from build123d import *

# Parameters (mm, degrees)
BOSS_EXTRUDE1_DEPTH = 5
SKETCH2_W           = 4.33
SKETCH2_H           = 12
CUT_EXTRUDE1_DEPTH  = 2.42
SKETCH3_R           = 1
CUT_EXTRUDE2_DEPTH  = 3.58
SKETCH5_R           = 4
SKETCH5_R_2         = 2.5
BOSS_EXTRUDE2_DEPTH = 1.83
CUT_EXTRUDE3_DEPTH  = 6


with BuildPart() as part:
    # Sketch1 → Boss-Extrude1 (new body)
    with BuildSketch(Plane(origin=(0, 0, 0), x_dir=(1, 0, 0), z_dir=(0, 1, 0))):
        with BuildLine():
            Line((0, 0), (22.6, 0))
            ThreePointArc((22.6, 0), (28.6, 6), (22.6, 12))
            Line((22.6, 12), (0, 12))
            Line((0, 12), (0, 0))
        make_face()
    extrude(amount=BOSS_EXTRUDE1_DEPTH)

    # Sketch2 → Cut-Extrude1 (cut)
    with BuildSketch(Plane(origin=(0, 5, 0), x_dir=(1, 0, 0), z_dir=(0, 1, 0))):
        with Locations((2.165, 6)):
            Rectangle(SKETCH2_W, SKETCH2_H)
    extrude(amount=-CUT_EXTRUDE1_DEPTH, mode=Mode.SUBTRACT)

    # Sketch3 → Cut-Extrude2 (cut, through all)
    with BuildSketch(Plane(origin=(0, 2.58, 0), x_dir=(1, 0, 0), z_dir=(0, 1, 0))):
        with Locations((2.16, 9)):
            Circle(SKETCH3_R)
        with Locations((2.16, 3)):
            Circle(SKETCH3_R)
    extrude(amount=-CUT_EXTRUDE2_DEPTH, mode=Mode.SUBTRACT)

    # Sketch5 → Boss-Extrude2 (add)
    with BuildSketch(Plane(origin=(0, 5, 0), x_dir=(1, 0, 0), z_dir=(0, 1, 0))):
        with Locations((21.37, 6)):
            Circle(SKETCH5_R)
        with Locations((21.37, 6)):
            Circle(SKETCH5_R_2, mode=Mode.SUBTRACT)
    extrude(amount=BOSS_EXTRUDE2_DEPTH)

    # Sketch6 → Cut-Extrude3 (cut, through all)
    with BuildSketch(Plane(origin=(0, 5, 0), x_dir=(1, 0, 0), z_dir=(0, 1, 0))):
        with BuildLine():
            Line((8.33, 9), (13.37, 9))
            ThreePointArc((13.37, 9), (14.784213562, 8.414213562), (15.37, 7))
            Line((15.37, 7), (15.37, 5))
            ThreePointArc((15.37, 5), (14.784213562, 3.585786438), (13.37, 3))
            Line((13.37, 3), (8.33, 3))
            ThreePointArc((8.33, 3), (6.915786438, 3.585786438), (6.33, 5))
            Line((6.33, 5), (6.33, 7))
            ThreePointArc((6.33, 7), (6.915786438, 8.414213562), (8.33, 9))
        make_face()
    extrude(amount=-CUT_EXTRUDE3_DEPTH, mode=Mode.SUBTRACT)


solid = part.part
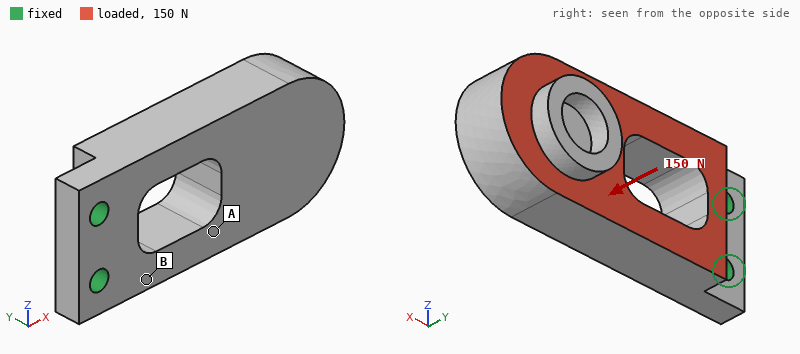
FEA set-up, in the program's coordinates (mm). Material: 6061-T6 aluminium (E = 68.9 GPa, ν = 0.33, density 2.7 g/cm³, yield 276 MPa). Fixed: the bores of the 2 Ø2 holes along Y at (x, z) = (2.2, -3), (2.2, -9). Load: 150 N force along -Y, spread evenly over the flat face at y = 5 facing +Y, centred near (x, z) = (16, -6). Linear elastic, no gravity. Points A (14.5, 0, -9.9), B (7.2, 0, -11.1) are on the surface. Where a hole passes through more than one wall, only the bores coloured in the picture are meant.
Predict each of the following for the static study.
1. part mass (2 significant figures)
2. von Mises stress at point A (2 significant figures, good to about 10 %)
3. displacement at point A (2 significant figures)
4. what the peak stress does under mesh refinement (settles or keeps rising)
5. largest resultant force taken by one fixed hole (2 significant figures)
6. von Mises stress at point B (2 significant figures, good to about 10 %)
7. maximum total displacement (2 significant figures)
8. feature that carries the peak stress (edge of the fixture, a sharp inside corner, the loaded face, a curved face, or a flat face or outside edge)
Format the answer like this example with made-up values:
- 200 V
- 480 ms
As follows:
- 3.5 g
- 20 MPa
- 0.063 mm
- keeps rising
- 76 N
- 56 MPa
- 0.16 mm
- edge of the fixture
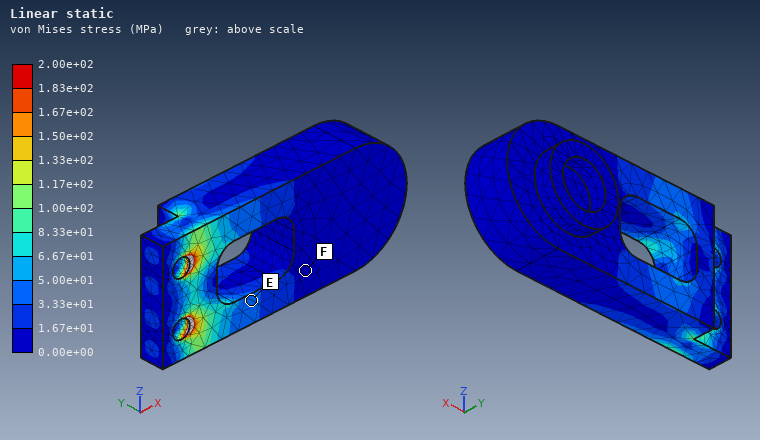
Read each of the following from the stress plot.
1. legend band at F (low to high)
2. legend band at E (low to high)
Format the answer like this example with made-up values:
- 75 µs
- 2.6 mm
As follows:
- 0.00e+00 to 1.67e+01 MPa
- 3.33e+01 to 5.00e+01 MPa
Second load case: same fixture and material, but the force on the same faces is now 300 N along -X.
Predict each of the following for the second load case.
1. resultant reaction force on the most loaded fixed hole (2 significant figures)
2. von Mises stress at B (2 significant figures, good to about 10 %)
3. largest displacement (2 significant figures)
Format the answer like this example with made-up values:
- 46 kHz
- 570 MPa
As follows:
- 150 N
- 22 MPa
- 98 µm
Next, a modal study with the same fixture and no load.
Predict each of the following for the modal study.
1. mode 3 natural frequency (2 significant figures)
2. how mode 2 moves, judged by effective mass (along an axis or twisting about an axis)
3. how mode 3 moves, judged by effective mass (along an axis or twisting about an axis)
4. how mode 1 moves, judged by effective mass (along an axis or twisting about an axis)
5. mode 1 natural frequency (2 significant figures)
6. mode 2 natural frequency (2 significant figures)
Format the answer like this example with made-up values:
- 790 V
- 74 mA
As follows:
- 14 kHz
- along Z
- twisting about X
- along Y
- 3100 Hz
- 7500 Hz
